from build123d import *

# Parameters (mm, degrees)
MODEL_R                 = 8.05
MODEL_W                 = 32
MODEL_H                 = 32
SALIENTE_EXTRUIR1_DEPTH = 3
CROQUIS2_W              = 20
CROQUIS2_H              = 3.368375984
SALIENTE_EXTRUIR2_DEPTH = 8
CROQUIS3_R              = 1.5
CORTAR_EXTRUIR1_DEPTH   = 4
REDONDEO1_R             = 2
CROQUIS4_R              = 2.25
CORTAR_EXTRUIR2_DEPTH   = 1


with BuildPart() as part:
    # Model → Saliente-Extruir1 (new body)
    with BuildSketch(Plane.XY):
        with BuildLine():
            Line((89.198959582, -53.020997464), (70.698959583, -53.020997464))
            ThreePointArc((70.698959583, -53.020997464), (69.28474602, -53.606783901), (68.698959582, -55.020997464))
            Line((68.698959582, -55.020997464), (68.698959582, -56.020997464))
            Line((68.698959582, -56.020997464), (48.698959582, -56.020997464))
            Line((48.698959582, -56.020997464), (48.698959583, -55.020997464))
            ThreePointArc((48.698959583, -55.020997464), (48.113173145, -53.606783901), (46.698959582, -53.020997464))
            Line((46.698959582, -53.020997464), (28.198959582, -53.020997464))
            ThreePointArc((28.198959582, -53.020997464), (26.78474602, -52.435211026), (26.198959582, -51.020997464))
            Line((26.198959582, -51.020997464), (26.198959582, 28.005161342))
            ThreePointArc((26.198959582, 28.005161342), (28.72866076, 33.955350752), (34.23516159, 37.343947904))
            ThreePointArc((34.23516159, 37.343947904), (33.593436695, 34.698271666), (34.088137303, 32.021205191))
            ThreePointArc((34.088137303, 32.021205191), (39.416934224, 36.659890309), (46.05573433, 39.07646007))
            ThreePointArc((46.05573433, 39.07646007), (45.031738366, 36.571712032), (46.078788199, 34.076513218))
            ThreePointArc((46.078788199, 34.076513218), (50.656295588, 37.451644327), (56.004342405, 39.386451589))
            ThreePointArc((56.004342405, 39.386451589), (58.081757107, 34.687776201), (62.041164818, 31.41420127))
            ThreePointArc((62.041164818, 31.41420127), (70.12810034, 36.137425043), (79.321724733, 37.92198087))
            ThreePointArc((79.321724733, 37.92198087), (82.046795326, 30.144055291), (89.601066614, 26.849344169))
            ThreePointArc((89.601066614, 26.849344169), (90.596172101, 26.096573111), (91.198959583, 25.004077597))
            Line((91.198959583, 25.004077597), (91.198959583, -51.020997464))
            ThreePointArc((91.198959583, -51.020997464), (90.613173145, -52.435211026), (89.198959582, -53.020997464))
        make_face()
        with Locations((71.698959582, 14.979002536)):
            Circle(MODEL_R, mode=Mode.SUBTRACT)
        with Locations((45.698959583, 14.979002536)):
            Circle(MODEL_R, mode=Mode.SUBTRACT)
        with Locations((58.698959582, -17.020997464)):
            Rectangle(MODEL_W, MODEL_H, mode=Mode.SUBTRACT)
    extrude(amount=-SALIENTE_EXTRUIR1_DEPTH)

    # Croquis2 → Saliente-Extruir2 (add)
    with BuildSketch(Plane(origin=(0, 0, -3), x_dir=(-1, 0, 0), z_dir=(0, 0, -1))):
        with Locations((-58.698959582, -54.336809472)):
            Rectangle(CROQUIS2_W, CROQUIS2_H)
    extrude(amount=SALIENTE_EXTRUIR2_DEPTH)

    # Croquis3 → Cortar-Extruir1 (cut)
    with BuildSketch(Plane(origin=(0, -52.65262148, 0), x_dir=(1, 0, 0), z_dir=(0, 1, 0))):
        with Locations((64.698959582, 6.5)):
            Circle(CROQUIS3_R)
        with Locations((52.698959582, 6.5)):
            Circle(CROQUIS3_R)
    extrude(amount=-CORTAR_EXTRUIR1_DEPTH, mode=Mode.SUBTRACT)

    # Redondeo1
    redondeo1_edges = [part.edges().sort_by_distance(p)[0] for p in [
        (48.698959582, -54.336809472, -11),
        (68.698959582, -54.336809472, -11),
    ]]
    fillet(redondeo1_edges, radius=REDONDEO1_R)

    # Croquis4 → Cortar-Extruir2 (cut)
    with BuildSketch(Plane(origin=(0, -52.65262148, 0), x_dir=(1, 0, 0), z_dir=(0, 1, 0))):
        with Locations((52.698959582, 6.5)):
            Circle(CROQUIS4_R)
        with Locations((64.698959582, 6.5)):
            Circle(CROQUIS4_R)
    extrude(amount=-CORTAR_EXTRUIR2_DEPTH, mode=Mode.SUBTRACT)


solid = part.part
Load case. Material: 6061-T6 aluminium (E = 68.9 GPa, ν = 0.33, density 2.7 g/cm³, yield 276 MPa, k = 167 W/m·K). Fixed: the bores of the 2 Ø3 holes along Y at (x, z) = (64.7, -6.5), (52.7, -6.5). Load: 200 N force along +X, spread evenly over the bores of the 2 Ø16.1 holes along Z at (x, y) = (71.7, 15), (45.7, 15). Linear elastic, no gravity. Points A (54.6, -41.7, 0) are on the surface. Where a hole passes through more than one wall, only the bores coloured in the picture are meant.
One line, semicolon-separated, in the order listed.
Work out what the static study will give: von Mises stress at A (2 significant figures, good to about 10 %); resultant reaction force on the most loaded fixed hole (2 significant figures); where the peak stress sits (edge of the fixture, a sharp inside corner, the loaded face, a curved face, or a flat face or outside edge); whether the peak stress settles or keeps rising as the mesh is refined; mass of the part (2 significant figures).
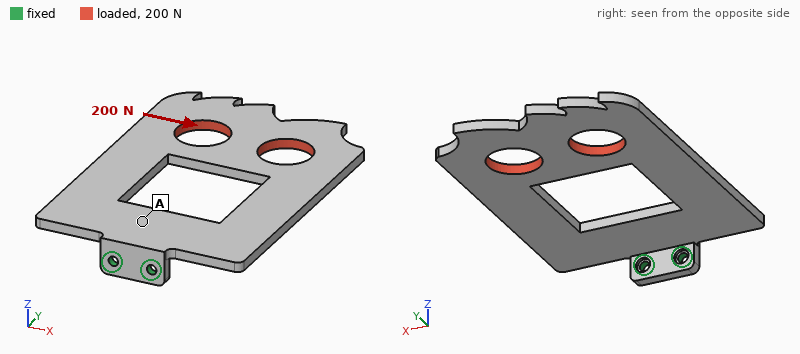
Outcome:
16 MPa; 1.0 kN; edge of the fixture; keeps rising; 36 g
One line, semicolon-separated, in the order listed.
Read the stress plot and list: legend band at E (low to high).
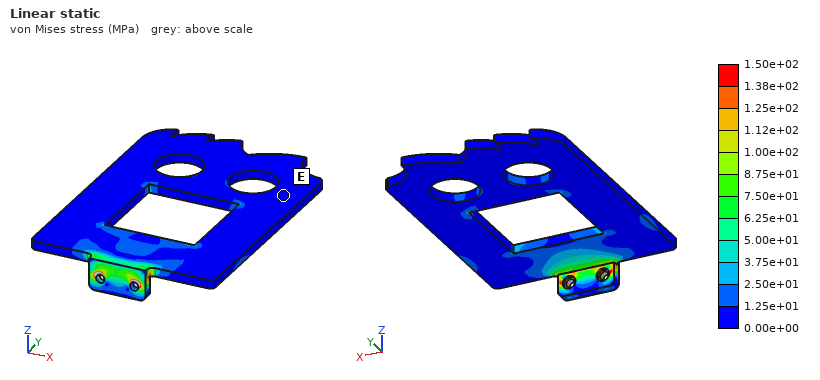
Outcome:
0.00e+00 to 1.25e+01 MPa
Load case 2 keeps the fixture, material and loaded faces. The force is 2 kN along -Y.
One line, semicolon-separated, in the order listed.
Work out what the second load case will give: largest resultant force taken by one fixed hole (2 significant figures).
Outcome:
1.0 kN
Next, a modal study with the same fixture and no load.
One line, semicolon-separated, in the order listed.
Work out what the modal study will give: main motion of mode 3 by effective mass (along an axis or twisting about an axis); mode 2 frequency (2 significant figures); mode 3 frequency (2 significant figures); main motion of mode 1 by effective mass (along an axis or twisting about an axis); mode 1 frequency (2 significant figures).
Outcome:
along X; 620 Hz; 910 Hz; along Z; 210 Hz
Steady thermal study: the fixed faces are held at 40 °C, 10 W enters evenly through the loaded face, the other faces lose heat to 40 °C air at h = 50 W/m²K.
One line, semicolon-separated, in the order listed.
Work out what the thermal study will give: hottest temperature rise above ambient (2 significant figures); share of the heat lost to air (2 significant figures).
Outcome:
23 K; 66 %
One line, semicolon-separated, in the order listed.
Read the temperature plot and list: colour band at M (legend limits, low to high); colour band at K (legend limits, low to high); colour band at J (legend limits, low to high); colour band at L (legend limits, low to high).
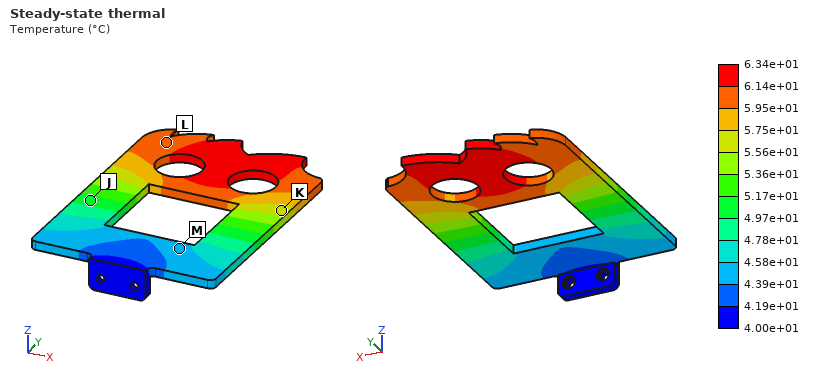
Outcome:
4.39e+01 to 4.58e+01 °C; 5.56e+01 to 5.75e+01 °C; 4.97e+01 to 5.17e+01 °C; 5.95e+01 to 6.14e+01 °C
